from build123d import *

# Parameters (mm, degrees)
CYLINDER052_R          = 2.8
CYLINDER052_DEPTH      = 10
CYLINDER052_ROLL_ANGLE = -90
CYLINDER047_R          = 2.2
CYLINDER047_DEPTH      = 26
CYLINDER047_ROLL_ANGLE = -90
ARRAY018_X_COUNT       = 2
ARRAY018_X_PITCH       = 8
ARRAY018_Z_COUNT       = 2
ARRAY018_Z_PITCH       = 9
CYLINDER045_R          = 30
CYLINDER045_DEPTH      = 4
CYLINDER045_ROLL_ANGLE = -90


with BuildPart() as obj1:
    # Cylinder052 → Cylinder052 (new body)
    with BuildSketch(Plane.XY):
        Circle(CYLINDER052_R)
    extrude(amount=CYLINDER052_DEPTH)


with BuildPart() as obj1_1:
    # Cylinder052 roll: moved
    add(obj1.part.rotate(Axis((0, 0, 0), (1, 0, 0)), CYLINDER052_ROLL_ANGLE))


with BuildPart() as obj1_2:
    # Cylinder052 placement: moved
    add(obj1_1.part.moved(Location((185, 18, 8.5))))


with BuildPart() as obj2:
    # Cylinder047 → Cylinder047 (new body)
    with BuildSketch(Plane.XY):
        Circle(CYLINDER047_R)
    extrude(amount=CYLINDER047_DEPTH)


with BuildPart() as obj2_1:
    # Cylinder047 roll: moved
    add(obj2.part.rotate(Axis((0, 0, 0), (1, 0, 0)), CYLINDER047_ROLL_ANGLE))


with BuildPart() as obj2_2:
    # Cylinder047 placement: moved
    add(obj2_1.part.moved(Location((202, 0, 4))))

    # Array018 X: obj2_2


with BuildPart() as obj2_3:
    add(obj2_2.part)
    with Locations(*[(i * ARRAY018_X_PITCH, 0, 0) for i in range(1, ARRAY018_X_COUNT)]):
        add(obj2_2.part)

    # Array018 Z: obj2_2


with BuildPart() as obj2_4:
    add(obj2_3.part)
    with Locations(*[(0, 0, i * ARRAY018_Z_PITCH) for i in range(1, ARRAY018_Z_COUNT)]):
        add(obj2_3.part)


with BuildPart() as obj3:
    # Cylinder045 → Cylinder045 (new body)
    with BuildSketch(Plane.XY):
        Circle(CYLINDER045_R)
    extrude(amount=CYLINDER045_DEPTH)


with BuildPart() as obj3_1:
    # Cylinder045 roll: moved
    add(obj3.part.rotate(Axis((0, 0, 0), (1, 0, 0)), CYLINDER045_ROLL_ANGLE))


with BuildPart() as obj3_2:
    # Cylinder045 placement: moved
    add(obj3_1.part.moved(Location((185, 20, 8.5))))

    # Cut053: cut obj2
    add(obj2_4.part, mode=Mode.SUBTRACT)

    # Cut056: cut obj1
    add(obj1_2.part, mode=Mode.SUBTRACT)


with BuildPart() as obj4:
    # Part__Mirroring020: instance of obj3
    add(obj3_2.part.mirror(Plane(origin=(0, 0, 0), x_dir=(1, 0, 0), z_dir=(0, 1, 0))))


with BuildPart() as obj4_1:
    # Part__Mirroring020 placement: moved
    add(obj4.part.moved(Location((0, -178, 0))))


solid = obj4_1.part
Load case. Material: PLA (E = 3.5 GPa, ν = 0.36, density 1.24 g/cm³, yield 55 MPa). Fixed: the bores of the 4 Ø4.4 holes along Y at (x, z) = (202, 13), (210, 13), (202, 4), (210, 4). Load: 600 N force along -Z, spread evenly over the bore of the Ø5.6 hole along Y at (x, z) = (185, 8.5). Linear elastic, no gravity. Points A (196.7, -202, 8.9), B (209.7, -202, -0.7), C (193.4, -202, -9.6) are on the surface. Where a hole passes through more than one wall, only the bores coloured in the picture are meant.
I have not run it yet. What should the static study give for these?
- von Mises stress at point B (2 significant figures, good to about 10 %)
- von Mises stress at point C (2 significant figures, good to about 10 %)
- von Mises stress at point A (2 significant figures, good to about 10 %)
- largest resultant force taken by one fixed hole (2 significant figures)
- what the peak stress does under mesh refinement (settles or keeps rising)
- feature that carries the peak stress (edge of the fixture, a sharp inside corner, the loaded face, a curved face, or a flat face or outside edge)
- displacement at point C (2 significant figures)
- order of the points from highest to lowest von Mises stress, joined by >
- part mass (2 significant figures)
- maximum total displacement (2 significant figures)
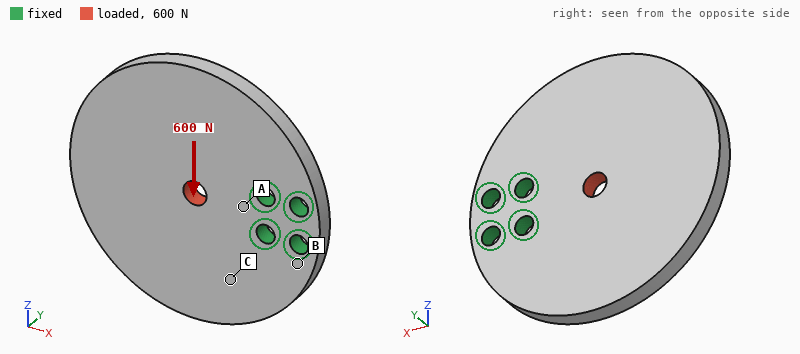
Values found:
8.7 MPa
3.1 MPa
17 MPa
610 N
keeps rising
edge of the fixture
0.100 mm
A > B > C
14 g
0.25 mm
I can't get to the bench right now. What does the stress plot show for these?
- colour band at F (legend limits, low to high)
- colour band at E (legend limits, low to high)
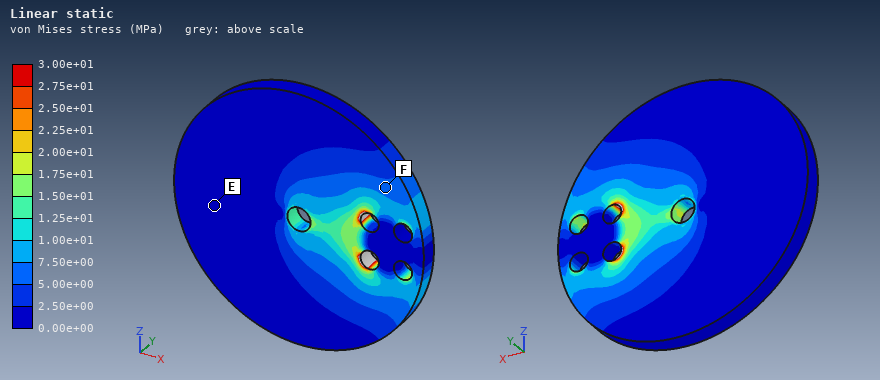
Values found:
5.00e+00 to 7.50e+00 MPa
0.00e+00 to 2.50e+00 MPa
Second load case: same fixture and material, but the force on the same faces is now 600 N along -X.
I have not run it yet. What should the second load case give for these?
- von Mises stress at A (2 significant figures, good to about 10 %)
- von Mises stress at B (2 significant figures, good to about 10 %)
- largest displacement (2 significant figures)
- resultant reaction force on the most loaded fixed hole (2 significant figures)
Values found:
6.2 MPa
2.0 MPa
44 µm
270 N
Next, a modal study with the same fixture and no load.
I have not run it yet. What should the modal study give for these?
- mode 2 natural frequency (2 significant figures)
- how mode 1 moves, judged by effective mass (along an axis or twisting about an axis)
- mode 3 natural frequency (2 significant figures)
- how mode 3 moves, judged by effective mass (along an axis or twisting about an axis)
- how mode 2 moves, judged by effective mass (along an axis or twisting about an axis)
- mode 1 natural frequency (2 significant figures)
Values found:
950 Hz
along Y
1900 Hz
along Y
twisting about X
550 Hz
